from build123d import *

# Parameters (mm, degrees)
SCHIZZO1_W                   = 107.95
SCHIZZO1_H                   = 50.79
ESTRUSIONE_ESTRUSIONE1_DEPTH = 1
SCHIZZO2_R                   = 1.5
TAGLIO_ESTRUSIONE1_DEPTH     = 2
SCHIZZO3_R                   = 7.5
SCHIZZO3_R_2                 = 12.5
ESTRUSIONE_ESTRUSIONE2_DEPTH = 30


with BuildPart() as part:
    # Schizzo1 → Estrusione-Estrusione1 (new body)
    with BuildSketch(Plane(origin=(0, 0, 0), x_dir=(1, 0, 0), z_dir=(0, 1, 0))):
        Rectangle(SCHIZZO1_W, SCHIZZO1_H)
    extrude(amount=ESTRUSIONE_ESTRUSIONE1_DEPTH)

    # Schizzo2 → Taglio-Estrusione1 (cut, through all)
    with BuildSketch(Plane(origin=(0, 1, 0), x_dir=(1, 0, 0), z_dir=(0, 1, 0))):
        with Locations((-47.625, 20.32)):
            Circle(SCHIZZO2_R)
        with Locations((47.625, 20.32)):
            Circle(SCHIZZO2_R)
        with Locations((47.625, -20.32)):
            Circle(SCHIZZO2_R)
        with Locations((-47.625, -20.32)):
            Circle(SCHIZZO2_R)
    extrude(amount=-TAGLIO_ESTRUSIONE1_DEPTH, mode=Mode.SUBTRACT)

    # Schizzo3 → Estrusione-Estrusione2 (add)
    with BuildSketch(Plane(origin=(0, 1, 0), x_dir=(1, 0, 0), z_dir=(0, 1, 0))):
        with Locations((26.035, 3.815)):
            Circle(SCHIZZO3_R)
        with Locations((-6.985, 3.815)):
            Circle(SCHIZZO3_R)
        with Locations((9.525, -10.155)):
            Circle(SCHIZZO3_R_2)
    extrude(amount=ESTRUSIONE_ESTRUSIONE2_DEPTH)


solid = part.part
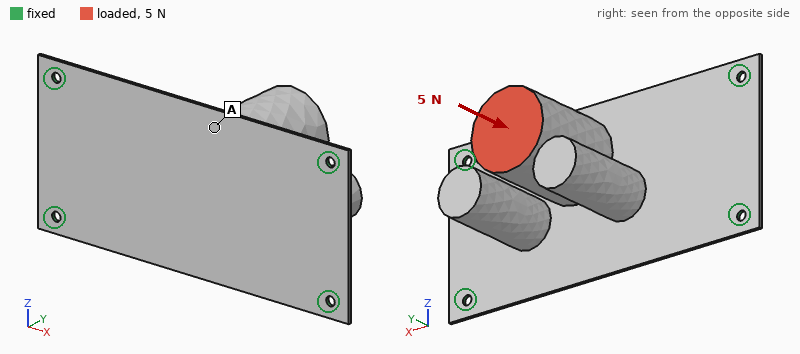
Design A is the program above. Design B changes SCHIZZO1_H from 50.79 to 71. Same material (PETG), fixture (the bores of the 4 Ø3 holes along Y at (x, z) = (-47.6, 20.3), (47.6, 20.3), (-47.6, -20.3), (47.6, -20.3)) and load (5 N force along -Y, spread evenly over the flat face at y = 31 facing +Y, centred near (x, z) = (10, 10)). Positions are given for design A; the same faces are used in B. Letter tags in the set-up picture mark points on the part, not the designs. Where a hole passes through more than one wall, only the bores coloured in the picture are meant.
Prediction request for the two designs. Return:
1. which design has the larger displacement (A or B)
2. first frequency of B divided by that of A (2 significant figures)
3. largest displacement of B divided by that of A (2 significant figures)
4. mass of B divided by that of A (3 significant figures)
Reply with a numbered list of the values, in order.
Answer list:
1. A
2. 1.1
3. 0.82
4. 1.07
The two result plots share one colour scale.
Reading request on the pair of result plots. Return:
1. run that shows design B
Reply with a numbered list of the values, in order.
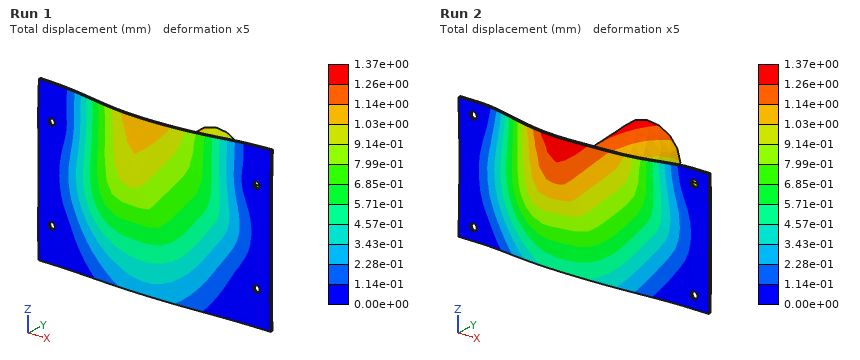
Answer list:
1. Run 1
